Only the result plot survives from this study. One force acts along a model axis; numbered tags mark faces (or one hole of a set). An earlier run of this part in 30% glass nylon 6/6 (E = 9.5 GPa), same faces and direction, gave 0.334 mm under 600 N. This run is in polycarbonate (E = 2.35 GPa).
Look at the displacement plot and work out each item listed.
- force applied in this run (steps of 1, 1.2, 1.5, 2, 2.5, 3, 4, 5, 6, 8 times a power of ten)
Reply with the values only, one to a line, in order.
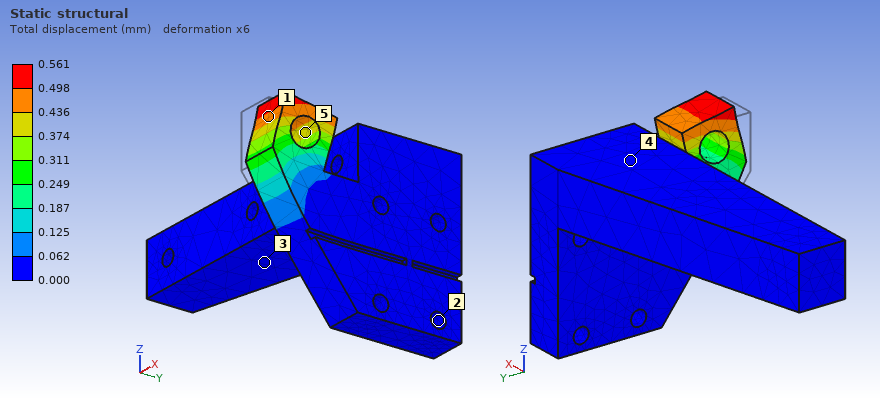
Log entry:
250 N
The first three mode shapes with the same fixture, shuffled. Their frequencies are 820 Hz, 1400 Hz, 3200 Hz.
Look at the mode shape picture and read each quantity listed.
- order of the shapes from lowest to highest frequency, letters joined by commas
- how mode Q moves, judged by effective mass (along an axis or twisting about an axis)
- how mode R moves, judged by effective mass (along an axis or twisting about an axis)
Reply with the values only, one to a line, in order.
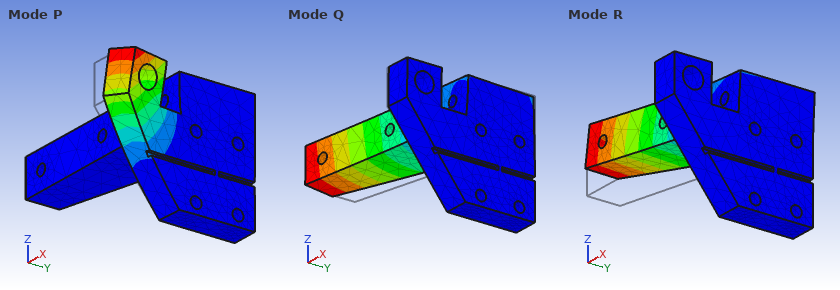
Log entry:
R, Q, P
along Y
along Z
